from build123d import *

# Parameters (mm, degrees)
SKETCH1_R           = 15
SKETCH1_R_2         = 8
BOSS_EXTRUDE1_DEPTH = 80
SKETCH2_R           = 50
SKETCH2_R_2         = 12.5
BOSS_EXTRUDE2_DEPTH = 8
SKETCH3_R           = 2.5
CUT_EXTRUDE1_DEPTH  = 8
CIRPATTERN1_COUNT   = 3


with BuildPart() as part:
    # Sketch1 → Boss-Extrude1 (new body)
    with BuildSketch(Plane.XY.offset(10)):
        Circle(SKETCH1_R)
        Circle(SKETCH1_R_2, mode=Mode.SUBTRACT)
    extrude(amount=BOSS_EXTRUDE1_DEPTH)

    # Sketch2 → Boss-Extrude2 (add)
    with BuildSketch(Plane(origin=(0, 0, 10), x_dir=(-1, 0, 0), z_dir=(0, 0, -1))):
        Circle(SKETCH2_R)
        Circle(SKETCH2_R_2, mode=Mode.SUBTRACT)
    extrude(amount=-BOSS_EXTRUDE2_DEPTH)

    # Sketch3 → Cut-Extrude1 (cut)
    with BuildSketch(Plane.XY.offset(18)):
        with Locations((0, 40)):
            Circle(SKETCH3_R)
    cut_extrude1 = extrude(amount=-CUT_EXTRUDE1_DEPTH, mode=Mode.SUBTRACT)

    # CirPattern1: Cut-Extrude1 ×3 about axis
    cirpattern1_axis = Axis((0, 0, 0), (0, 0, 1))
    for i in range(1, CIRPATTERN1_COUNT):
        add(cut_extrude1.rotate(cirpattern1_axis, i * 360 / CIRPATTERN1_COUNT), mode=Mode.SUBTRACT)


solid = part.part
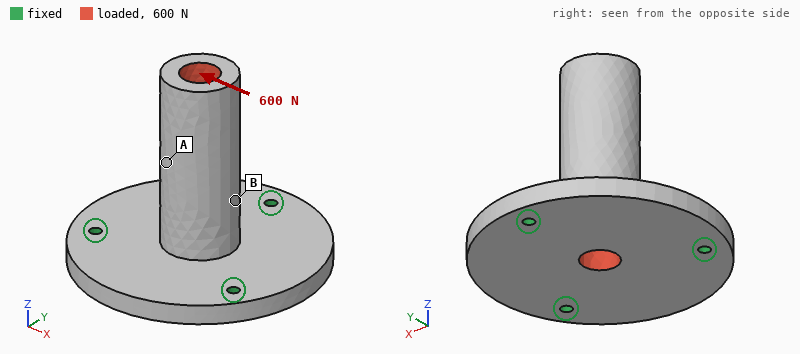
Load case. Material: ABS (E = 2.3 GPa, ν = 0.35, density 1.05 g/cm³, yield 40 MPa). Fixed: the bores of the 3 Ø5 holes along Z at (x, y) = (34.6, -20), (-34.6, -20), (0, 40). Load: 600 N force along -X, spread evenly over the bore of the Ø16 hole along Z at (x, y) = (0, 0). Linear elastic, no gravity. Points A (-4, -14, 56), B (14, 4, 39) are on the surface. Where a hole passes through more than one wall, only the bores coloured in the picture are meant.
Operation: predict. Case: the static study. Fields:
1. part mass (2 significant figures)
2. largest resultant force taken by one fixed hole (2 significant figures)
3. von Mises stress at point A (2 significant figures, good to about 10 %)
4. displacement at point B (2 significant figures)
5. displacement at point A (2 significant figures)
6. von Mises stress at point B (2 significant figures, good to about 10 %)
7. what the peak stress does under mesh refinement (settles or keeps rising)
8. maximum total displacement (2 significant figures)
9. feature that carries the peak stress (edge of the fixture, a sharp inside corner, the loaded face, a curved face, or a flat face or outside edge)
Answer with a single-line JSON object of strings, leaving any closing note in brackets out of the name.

{"part mass": "100 g", "largest resultant force taken by one fixed hole": "390 N", "von Mises stress at point A": "1.3 MPa", "displacement at point B": "0.46 mm", "displacement at point A": "0.71 mm", "von Mises stress at point B": "3.7 MPa", "what the peak stress does under mesh refinement": "keeps rising", "maximum total displacement": "1.4 mm", "feature that carries the peak stress": "edge of the fixture"}
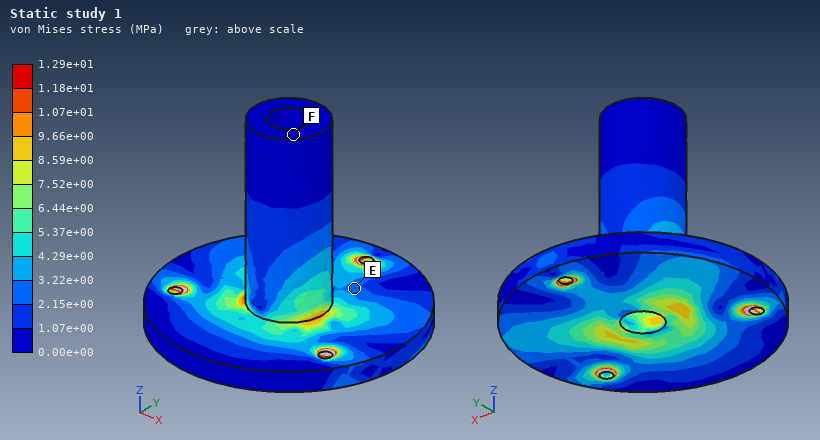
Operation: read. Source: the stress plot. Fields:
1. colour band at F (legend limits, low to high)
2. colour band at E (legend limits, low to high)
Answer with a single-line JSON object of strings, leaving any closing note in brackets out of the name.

{"colour band at F": "0.00e+00 to 1.07e+00 MPa", "colour band at E": "2.15e+00 to 3.22e+00 MPa"}
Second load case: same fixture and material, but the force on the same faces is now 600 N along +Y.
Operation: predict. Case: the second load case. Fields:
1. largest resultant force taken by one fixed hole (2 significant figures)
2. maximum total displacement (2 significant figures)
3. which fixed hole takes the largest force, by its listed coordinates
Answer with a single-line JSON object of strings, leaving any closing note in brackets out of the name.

{"largest resultant force taken by one fixed hole": "450 N", "maximum total displacement": "1.4 mm", "which fixed hole takes the largest force, by its listed coordinates": "(0, 40)"}
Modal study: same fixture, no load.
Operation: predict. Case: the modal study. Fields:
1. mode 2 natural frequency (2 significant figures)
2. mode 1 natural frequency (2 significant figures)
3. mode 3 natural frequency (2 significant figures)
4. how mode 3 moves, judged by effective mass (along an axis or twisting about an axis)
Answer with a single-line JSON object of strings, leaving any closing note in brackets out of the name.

{"mode 2 natural frequency": "610 Hz", "mode 1 natural frequency": "610 Hz", "mode 3 natural frequency": "1300 Hz", "how mode 3 moves, judged by effective mass": "along Z"}
